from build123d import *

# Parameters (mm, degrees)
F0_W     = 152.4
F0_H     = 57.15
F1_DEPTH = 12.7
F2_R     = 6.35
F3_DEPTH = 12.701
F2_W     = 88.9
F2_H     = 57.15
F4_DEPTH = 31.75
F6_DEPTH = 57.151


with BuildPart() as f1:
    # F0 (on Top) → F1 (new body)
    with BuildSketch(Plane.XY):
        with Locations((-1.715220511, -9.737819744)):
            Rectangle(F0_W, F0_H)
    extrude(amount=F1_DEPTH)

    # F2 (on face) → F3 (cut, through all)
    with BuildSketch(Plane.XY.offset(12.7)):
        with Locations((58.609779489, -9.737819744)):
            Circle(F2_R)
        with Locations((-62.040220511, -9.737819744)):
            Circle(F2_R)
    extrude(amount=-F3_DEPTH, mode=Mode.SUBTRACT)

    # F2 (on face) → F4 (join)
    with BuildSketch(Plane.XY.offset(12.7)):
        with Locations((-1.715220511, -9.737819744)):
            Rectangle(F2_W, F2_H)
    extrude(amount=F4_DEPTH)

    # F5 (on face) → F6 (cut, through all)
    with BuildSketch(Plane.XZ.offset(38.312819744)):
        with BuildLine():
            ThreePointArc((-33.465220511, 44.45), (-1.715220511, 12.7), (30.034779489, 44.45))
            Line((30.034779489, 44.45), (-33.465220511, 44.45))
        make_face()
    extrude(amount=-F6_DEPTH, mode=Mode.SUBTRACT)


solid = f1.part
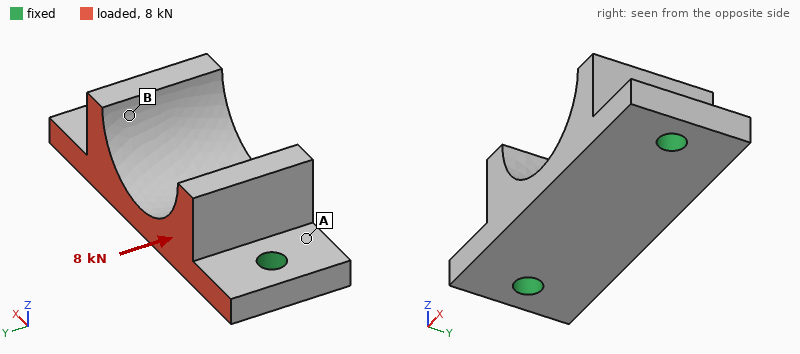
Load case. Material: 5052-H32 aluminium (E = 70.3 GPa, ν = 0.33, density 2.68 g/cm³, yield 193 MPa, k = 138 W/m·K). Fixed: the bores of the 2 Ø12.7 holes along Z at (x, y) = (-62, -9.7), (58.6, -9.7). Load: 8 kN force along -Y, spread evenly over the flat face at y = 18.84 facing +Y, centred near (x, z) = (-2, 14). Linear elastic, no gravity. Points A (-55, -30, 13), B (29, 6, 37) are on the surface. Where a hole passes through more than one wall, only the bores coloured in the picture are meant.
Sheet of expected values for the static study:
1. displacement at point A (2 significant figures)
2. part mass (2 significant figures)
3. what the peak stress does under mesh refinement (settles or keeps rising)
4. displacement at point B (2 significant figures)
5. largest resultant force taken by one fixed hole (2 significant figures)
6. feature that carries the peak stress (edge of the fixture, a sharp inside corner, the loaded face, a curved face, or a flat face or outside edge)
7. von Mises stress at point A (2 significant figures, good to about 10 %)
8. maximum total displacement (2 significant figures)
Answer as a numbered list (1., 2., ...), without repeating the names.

1. 7.8 µm
2. 480 g
3. keeps rising
4. 25 µm
5. 4.0 kN
6. edge of the fixture
7. 10.0 MPa
8. 32 µm
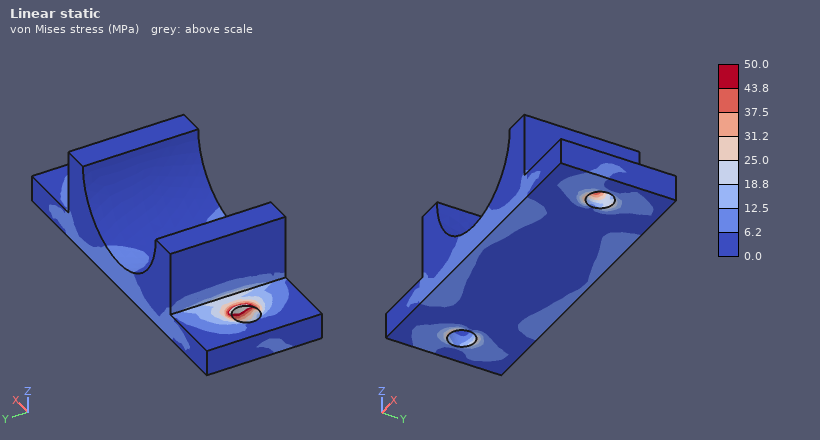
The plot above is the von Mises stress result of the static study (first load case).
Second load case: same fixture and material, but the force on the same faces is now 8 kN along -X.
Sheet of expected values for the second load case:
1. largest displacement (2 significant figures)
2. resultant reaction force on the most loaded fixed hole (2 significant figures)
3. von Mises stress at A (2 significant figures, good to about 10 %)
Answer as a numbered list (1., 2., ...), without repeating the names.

1. 15 µm
2. 4.4 kN
3. 2.2 MPa
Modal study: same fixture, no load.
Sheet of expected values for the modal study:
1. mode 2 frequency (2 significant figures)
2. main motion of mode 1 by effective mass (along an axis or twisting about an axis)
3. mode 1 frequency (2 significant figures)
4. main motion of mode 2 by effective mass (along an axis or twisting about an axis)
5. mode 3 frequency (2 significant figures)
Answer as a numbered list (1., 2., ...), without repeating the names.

1. 3800 Hz
2. along Z
3. 3400 Hz
4. along Y
5. 6400 Hz
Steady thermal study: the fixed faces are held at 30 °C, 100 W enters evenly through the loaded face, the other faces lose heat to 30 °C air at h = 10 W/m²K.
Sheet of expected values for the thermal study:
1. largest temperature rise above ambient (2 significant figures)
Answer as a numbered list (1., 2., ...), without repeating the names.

1. 17 K
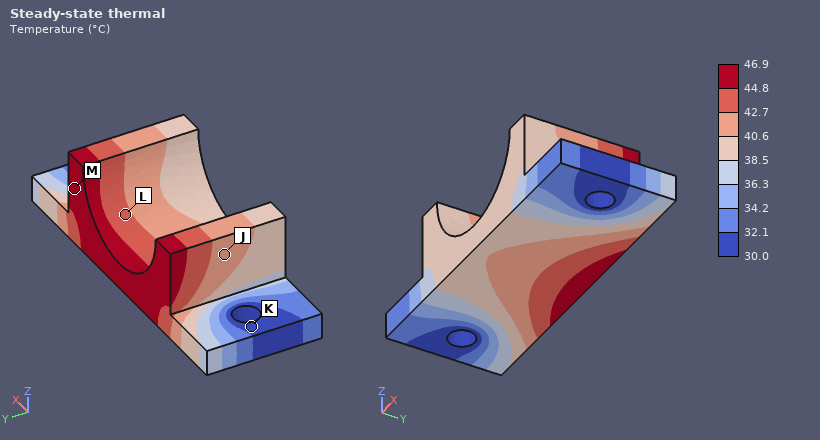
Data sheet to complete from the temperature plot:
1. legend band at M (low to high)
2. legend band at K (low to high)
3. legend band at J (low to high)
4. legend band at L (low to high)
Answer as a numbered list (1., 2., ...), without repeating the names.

1. 44.8 to 46.9 °C
2. 30.0 to 32.1 °C
3. 40.6 to 42.7 °C
4. 42.7 to 44.8 °C
